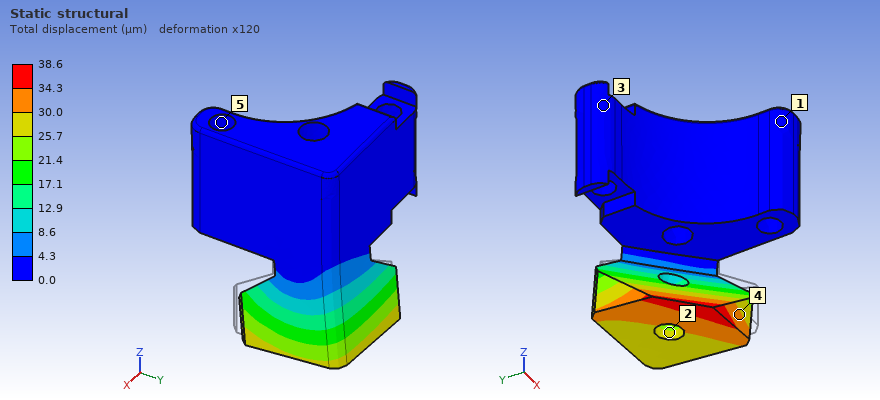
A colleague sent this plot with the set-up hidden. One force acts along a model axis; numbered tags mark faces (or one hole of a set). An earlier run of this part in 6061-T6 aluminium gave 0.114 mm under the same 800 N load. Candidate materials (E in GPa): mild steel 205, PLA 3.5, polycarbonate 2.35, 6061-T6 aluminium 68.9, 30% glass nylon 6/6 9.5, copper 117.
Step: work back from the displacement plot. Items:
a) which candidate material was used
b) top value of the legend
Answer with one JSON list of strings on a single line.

["mild steel", "38.6 µm"]
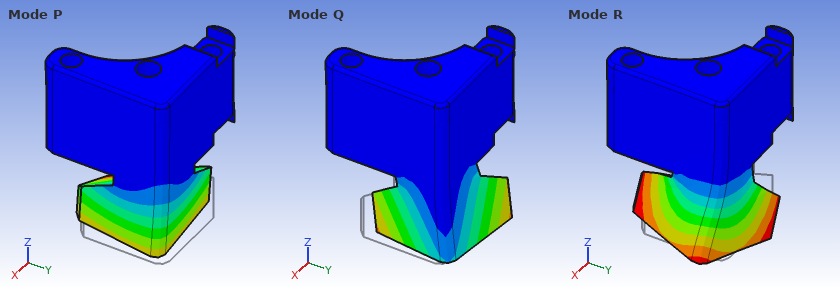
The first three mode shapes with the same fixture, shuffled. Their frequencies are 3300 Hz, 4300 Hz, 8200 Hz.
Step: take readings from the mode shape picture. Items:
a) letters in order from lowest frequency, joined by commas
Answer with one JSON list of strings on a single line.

["P, Q, R"]
